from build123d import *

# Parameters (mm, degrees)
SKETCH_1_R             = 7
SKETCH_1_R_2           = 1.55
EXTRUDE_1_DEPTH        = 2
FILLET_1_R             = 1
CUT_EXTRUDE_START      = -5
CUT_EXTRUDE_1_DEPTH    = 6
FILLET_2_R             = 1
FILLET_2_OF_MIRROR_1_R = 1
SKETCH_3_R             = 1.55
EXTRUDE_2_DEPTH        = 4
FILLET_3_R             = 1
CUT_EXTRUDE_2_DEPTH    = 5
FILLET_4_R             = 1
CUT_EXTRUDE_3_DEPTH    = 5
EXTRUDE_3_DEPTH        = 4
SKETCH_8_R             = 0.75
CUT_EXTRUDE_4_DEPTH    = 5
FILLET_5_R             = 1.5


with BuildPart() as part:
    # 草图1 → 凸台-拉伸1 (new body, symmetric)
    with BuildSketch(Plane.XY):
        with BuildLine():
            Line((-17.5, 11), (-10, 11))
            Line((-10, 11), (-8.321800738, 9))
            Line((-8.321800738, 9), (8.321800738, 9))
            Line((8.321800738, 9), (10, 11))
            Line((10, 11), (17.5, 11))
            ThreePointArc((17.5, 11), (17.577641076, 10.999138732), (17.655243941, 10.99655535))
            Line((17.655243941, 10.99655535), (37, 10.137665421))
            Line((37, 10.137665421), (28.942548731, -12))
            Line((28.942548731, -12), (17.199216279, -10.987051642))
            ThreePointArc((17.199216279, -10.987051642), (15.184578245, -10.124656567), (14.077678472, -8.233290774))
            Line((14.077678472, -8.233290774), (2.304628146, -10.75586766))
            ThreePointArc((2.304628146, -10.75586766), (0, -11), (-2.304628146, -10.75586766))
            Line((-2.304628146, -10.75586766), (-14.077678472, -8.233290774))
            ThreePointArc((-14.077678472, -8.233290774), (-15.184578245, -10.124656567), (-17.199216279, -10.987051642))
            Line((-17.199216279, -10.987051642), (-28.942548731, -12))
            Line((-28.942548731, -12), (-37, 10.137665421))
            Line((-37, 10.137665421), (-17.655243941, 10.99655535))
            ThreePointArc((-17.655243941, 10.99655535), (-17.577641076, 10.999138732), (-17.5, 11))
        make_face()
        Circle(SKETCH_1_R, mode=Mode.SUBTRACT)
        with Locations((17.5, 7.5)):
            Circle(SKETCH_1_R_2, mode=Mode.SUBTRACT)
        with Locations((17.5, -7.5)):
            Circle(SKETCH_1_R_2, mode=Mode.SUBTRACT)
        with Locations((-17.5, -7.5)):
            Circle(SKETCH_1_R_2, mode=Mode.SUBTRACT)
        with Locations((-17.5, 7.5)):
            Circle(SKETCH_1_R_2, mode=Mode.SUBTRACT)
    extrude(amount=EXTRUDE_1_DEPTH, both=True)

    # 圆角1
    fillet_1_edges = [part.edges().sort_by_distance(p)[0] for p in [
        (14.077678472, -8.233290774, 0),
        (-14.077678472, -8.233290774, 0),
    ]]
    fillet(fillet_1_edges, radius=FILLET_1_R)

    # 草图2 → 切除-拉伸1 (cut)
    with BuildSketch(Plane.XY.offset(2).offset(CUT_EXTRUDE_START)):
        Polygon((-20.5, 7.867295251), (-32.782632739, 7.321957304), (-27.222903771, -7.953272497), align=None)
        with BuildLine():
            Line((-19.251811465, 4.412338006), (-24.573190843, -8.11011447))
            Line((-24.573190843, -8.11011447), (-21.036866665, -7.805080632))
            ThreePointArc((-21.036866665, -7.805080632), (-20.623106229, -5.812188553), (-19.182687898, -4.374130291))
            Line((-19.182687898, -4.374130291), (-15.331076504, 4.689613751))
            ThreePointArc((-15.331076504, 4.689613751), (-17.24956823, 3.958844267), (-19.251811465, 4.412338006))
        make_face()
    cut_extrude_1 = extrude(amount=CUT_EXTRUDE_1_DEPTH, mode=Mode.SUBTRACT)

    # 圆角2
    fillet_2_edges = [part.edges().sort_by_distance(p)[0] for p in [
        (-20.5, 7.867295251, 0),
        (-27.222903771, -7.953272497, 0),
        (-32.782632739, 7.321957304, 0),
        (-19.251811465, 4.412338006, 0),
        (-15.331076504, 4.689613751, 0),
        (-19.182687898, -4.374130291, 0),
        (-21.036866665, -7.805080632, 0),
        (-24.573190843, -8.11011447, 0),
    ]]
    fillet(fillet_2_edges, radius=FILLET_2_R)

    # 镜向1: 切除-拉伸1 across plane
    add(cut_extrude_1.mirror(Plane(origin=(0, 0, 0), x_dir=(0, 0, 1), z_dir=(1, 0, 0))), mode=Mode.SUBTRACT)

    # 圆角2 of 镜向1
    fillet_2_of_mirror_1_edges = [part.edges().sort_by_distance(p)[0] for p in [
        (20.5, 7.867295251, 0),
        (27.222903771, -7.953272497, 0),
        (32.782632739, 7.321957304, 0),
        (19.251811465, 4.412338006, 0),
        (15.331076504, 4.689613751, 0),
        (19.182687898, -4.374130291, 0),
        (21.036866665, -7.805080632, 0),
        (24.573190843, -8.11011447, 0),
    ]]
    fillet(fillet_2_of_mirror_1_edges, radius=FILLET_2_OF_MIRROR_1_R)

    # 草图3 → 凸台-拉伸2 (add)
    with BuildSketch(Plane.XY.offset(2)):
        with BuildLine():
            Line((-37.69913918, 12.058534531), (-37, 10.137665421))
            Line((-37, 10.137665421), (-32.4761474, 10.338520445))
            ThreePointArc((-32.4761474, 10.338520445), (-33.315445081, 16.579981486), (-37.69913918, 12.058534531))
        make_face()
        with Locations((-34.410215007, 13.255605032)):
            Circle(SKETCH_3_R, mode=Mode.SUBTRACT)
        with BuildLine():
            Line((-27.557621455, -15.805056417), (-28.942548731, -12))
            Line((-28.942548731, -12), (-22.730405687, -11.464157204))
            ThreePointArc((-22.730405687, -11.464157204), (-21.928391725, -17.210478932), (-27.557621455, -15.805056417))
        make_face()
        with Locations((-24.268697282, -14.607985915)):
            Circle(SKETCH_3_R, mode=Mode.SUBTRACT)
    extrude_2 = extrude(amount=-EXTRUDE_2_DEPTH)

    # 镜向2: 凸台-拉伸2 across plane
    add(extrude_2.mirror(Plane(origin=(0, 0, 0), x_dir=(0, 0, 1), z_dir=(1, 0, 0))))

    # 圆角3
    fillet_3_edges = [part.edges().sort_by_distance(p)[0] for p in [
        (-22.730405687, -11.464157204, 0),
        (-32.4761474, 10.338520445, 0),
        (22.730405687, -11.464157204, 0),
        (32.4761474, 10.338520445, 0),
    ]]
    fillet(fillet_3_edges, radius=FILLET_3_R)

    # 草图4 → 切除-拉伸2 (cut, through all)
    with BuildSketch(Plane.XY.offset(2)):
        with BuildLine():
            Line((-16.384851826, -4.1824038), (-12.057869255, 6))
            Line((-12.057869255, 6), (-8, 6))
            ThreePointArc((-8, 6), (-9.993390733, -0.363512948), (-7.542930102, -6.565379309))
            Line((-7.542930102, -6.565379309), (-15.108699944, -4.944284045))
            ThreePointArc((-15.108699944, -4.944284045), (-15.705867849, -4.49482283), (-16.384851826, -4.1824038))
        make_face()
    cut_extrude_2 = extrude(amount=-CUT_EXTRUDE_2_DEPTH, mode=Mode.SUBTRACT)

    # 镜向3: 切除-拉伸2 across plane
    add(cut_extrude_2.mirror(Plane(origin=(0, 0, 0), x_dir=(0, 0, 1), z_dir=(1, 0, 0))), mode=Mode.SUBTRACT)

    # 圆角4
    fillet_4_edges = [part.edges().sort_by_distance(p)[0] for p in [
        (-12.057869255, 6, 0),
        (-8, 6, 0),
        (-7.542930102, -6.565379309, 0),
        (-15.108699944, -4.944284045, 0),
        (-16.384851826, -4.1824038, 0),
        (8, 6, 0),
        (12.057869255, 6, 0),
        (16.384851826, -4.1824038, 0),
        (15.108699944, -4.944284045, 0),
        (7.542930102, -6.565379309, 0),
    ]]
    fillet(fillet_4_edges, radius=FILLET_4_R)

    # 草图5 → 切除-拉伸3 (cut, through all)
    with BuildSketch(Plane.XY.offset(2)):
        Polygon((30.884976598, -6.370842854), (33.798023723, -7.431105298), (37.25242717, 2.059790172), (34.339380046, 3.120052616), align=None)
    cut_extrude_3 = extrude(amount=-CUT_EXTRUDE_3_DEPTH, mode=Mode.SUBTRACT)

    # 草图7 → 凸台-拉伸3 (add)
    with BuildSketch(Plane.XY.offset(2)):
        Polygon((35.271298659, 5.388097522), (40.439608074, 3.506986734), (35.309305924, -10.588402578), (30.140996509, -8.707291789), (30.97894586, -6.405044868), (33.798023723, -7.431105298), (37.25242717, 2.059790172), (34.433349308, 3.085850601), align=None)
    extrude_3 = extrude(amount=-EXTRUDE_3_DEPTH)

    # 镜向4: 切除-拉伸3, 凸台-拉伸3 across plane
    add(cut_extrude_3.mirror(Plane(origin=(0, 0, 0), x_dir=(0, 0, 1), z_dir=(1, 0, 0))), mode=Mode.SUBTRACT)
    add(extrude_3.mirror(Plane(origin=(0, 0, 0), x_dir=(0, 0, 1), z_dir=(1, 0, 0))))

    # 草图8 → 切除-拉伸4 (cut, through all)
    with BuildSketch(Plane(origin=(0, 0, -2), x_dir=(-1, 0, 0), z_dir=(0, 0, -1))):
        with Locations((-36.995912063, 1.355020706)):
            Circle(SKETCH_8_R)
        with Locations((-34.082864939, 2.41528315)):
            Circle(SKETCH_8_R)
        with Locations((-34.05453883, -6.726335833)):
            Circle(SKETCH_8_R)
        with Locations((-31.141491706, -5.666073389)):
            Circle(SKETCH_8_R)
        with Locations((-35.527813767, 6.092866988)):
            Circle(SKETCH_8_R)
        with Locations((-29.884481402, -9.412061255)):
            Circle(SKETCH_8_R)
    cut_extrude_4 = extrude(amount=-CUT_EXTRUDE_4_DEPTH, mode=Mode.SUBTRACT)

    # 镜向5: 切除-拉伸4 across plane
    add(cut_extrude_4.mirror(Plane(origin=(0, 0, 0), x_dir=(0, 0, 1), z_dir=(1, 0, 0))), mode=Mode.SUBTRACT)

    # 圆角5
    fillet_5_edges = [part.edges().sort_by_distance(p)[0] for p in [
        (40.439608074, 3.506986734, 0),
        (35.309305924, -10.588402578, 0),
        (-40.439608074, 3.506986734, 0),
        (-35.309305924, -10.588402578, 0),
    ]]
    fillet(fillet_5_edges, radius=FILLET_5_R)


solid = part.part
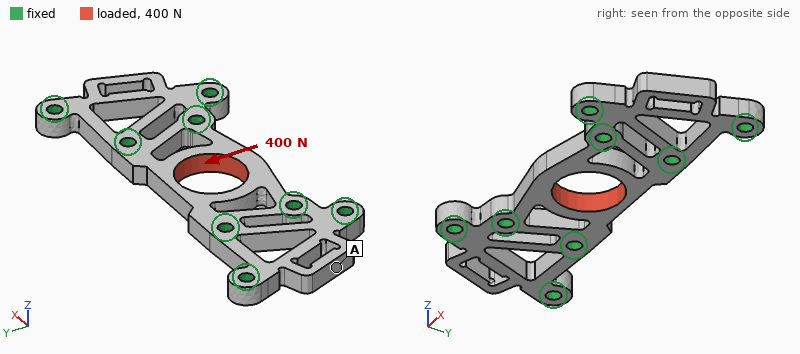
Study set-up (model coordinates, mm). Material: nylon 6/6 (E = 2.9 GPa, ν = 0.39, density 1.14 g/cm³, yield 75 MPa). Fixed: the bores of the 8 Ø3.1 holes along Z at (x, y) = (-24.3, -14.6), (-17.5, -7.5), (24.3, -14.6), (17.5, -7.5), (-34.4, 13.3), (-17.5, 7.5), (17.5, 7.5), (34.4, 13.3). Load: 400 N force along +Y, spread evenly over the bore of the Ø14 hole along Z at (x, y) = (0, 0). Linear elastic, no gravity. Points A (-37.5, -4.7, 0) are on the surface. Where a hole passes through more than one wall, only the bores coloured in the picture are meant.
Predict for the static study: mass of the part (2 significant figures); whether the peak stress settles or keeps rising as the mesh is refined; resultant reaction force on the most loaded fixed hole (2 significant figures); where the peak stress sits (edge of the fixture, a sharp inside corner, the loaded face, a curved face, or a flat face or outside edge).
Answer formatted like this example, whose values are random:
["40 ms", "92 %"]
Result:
["4.7 g", "keeps rising", "140 N", "a sharp inside corner"]
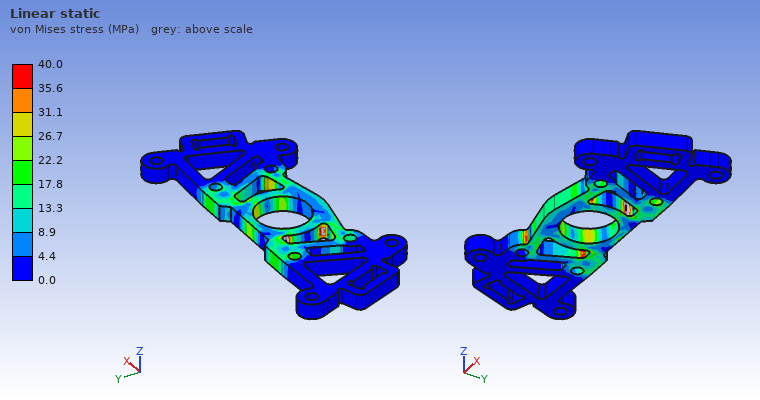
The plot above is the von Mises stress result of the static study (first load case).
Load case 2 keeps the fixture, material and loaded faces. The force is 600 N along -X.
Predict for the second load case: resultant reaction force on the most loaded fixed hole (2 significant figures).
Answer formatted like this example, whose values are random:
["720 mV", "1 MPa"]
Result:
["150 N"]
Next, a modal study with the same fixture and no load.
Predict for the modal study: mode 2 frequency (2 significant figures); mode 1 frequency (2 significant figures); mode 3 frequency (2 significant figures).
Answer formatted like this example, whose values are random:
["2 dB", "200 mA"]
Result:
["4900 Hz", "4900 Hz", "5000 Hz"]
